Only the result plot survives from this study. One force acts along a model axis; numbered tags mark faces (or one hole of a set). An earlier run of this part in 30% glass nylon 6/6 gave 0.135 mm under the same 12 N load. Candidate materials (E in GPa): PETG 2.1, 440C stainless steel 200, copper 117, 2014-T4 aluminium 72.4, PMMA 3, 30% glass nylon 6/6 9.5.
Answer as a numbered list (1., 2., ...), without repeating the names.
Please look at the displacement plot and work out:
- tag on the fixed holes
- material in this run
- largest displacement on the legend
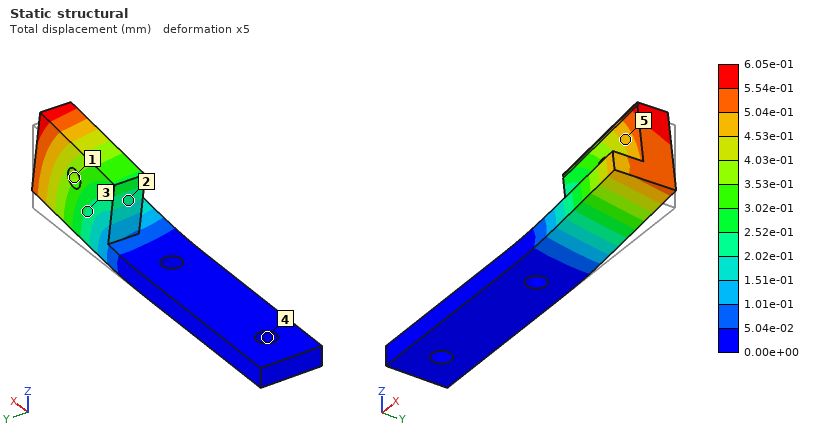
1. 4
2. PETG
3. 6.05e-01 mm
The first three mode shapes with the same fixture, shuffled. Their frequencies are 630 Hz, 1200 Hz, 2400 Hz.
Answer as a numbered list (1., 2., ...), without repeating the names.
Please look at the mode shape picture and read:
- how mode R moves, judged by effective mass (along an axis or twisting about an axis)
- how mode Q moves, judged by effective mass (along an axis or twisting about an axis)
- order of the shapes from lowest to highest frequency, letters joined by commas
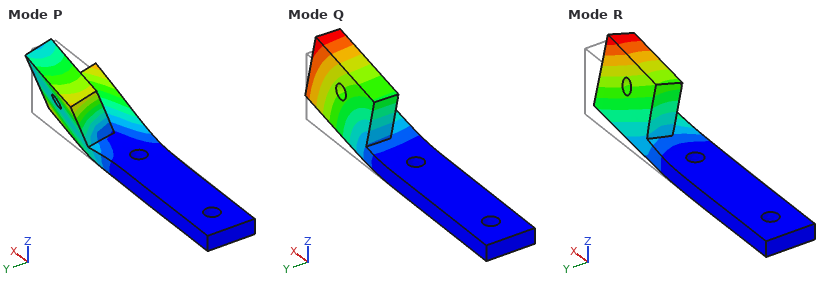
1. along Y
2. along Z
3. Q, R, P
